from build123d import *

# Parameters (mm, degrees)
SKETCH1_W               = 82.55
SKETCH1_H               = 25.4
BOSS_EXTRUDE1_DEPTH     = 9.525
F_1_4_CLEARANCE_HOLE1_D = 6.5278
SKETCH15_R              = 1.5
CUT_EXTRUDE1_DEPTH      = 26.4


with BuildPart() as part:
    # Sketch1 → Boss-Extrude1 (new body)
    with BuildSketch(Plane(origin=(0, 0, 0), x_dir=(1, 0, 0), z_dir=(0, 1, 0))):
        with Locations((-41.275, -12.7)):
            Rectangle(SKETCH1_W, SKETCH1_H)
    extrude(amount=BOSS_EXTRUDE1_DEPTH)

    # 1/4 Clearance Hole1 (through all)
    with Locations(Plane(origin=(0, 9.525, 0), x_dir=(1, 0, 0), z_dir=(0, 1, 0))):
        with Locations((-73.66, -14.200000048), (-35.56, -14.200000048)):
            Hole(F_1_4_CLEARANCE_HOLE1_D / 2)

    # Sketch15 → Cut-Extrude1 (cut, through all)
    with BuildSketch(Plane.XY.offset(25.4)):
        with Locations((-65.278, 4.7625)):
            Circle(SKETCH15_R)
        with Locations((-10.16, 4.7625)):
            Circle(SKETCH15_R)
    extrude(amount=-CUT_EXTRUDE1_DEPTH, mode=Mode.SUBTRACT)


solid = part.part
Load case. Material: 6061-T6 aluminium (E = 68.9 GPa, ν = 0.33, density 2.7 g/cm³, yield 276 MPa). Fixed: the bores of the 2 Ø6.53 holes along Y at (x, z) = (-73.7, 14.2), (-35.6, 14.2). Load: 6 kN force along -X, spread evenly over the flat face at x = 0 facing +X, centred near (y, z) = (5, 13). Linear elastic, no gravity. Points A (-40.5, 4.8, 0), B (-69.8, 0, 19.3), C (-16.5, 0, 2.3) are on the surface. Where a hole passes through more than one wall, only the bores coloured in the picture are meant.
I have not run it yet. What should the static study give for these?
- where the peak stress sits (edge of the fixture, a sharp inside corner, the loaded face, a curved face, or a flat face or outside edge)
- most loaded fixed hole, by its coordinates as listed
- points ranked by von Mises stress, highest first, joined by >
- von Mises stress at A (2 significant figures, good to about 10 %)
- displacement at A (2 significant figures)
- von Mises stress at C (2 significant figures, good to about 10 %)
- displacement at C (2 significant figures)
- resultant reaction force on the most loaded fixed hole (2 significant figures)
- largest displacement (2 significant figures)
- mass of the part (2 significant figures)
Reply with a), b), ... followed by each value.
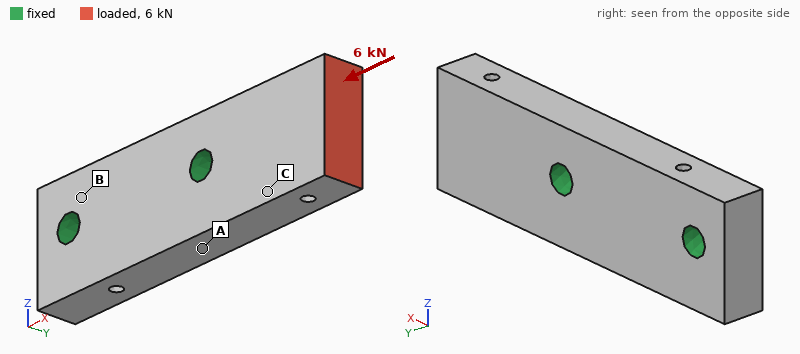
a) a curved face
b) (-35.6, 14.2)
c) C > A > B
d) 15 MPa
e) 3.2 µm
f) 27 MPa
g) 10 µm
h) 5.4 kN
i) 17 µm
j) 51 g
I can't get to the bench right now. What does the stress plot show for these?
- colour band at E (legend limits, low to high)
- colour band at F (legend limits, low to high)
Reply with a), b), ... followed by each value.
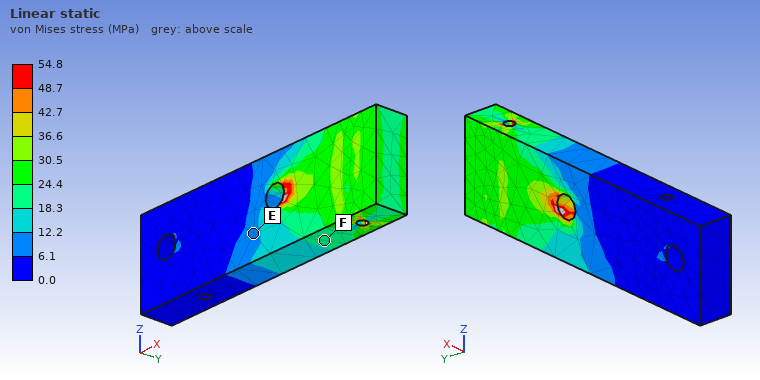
a) 6.1 to 12.2 MPa
b) 18.3 to 24.4 MPa
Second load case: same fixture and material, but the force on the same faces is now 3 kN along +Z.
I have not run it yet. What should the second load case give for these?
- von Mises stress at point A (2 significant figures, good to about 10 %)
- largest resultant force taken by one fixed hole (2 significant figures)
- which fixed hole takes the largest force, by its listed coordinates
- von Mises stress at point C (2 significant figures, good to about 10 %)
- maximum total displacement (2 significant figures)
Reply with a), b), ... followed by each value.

a) 66 MPa
b) 4.7 kN
c) (-35.6, 14.2)
d) 45 MPa
e) 0.12 mm
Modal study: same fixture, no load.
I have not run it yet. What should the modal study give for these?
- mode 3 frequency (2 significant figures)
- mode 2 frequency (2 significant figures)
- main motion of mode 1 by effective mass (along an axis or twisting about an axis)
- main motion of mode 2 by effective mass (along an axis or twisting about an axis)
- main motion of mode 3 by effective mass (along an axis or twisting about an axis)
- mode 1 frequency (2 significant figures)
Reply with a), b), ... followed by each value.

a) 14 kHz
b) 9700 Hz
c) along Y
d) along Z
e) twisting about X
f) 6000 Hz
